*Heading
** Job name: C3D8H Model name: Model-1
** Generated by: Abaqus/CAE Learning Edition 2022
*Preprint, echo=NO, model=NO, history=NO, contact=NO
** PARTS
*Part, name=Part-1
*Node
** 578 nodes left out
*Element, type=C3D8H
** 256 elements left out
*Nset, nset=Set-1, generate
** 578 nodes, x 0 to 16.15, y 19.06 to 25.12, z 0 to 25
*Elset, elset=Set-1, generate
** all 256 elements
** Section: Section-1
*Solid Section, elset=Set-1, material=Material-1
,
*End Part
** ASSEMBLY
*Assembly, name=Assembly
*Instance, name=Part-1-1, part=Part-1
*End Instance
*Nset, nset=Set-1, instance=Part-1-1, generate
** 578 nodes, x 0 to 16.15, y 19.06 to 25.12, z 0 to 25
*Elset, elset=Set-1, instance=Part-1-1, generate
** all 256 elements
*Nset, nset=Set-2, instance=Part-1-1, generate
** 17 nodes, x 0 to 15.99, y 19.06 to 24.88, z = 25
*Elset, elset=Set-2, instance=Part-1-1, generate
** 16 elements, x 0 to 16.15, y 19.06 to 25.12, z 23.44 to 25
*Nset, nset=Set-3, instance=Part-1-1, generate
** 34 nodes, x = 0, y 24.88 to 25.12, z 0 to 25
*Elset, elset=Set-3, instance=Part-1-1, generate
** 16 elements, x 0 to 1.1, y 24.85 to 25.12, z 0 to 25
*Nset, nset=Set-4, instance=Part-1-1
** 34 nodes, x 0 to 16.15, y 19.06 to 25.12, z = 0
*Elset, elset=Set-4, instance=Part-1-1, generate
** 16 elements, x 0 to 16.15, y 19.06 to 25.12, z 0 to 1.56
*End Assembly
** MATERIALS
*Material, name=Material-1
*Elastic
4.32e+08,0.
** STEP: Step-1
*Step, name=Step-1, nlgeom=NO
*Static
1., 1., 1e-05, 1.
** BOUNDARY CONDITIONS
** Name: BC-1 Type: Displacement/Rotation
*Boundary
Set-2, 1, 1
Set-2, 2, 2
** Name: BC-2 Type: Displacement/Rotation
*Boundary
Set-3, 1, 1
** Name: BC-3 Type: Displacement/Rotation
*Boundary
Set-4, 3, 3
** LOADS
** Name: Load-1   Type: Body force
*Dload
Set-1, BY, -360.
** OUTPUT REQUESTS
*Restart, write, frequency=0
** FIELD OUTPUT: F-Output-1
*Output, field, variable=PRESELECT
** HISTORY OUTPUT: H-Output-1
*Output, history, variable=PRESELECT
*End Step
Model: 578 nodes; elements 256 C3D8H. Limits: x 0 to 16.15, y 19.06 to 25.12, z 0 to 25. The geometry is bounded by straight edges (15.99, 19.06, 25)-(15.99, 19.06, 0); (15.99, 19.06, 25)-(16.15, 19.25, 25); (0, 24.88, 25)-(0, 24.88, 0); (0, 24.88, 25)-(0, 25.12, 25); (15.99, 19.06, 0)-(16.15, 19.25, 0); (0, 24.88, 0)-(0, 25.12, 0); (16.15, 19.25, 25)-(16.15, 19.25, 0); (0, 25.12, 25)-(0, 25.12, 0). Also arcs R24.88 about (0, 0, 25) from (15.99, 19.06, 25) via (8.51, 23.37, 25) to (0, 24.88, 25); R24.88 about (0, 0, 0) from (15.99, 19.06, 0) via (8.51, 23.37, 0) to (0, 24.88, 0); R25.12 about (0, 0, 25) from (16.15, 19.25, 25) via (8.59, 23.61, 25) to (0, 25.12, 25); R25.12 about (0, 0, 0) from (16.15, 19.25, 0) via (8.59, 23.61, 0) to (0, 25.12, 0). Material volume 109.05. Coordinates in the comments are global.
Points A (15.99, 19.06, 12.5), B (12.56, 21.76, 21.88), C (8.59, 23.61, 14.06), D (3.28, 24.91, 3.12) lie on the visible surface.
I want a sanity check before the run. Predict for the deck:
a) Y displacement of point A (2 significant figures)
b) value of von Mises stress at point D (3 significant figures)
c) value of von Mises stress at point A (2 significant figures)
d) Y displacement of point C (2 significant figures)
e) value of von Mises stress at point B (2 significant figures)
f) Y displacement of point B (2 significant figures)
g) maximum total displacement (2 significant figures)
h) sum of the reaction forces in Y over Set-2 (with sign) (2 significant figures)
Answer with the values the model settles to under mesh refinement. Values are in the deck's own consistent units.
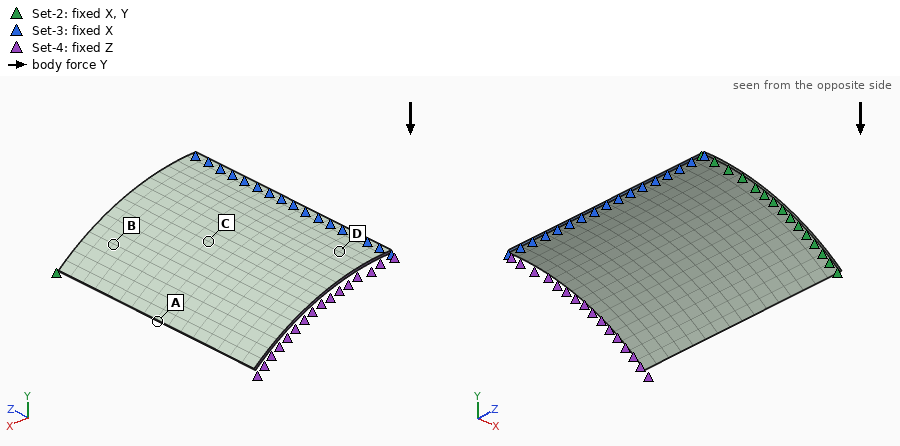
-0.22
1.75e+05
3.2e+05
-0.051
2.7e+05
-0.041
0.34
39000
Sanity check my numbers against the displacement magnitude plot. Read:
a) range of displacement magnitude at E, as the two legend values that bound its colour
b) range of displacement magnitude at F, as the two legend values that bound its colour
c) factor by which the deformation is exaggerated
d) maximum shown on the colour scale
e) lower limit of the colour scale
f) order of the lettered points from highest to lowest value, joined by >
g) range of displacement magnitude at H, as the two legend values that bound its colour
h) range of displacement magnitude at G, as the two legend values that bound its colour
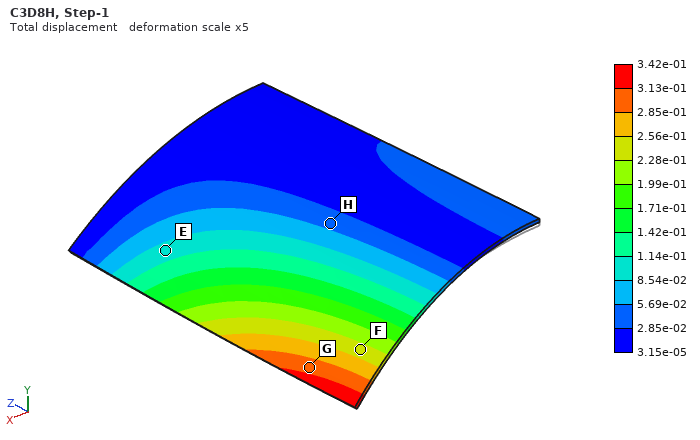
8.54e-02 to 1.14e-01
2.28e-01 to 2.56e-01
5
3.42e-01
3.15e-05
G > F > E > H
2.85e-02 to 5.69e-02
2.85e-01 to 3.13e-01
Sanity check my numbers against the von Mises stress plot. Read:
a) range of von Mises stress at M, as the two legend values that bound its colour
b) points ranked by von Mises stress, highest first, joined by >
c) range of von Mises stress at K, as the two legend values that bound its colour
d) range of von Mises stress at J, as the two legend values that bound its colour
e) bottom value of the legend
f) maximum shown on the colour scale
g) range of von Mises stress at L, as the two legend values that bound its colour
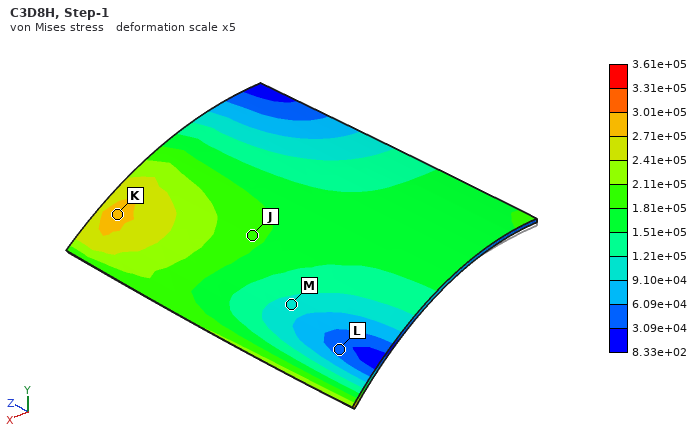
9.10e+04 to 1.21e+05
K > J > M > L
2.71e+05 to 3.01e+05
1.81e+05 to 2.11e+05
8.33e+02
3.61e+05
3.09e+04 to 6.09e+04
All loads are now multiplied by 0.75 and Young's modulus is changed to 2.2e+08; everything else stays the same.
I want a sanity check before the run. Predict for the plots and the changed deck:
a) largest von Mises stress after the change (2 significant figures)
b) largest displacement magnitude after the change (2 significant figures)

2.7e+05
0.50
